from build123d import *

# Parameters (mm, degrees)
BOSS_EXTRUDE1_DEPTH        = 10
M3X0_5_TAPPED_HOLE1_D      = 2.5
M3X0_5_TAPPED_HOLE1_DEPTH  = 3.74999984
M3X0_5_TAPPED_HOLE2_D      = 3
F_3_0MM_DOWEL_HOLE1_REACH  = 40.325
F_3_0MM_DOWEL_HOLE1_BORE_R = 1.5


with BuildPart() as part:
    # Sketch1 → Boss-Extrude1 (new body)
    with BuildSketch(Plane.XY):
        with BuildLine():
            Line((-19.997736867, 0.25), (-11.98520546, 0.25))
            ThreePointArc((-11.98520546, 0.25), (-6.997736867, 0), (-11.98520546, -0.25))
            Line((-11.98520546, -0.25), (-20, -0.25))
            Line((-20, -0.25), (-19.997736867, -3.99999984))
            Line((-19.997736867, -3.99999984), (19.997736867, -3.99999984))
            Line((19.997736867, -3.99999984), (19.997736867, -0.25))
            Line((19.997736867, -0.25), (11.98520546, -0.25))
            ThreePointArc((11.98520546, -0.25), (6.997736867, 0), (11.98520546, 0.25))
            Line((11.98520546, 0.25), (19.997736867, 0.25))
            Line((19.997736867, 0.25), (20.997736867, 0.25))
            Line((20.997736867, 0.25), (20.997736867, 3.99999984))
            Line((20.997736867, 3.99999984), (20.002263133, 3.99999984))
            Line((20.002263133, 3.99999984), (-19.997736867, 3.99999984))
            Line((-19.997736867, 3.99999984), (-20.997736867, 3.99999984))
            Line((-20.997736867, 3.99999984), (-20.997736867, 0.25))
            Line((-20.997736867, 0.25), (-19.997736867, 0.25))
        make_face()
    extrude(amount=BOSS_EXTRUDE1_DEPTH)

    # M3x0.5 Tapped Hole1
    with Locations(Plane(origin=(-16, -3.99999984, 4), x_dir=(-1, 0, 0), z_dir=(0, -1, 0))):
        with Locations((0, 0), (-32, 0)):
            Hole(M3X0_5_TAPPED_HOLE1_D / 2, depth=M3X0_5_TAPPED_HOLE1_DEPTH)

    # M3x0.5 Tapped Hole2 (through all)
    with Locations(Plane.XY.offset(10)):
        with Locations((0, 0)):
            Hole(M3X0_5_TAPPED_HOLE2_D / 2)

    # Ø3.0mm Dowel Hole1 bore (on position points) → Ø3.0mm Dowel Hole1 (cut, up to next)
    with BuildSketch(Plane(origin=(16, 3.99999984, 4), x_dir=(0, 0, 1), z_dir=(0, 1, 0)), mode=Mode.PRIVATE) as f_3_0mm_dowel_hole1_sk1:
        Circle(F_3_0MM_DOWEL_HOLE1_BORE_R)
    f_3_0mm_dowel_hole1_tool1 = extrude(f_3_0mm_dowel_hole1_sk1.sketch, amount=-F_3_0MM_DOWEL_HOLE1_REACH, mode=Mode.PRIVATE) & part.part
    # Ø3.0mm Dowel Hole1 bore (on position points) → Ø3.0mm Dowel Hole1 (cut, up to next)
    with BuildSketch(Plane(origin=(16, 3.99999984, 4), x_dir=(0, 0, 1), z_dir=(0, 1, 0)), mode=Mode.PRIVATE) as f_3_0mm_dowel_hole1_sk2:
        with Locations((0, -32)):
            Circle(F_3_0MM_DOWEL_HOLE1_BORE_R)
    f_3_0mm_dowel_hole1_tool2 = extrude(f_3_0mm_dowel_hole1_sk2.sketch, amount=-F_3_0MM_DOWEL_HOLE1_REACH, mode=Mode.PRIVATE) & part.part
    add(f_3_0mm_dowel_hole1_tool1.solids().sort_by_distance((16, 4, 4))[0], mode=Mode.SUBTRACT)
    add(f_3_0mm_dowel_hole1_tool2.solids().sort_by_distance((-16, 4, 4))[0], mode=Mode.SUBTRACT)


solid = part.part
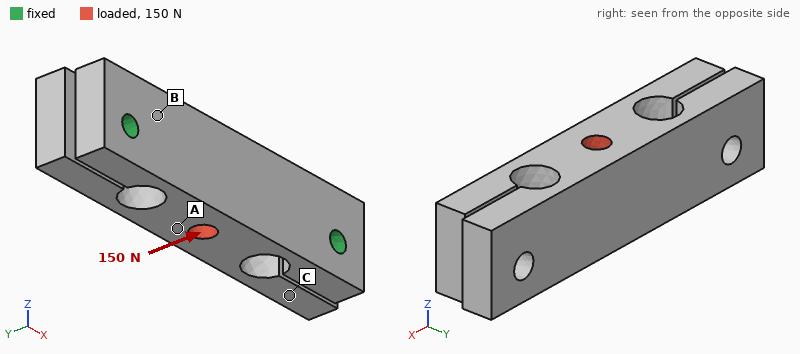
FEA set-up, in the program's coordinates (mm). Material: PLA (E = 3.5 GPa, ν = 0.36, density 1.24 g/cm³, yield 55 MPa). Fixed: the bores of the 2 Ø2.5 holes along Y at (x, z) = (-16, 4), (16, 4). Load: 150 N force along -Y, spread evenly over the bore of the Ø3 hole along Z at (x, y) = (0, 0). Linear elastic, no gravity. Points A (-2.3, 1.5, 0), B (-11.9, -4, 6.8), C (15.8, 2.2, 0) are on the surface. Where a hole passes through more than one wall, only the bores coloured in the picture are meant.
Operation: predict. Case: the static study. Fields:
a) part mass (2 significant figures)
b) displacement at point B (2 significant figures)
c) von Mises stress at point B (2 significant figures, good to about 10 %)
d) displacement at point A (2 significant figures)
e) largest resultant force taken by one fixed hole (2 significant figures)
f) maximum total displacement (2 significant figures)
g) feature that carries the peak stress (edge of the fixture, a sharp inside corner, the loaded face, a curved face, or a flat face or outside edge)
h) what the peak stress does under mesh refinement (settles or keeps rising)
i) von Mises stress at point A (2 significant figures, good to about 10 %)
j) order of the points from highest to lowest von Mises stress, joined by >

3.3 g
0.041 mm
13 MPa
0.12 mm
75 N
0.15 mm
edge of the fixture
keeps rising
4.6 MPa
B > A > C
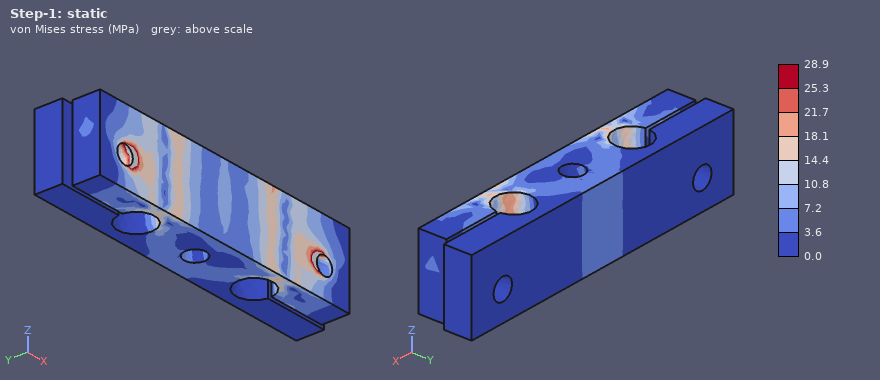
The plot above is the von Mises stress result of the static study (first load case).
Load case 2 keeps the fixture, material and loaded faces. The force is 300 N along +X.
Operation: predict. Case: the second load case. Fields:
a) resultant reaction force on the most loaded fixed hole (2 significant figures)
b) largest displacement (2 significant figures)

160 N
0.19 mm
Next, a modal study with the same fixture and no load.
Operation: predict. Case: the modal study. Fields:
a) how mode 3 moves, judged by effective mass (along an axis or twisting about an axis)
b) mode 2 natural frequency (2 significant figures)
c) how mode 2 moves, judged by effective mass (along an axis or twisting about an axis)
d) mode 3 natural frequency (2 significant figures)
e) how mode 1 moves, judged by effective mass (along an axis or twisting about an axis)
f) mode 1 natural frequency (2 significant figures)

along Z
1700 Hz
along Y
2200 Hz
twisting about Z
1600 Hz
